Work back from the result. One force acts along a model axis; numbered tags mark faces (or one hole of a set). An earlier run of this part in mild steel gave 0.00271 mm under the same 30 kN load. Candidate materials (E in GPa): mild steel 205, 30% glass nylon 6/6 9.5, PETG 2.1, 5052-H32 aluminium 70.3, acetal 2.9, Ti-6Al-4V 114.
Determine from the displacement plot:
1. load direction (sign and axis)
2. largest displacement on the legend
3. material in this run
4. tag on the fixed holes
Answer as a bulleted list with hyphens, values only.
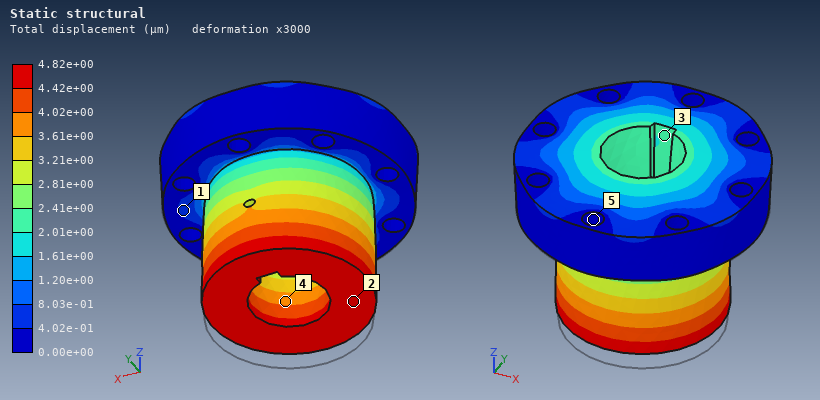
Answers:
- +Z
- 4.82e+00 µm
- Ti-6Al-4V
- 5
